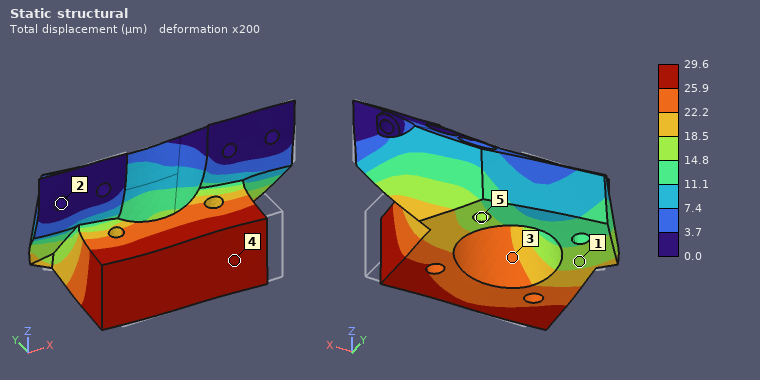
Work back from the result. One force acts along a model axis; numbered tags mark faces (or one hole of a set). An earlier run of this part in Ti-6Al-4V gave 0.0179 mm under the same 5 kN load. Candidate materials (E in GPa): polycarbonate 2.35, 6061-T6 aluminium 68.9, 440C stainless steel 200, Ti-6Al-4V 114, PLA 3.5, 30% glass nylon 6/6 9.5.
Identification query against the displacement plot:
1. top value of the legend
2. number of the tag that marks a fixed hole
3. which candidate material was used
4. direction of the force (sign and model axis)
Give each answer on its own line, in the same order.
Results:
29.6 µm
2
6061-T6 aluminium
-X
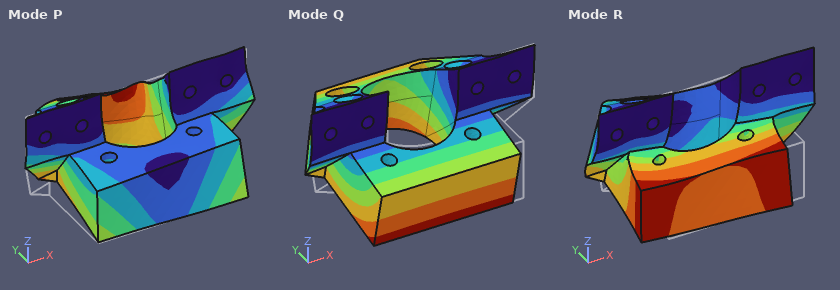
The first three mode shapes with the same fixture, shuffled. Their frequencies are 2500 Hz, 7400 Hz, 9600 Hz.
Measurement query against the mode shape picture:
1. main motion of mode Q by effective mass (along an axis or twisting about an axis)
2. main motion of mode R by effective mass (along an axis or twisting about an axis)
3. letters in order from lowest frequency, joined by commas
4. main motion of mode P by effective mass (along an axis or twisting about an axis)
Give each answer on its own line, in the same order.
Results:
along Y
along X
Q, R, P
along X
